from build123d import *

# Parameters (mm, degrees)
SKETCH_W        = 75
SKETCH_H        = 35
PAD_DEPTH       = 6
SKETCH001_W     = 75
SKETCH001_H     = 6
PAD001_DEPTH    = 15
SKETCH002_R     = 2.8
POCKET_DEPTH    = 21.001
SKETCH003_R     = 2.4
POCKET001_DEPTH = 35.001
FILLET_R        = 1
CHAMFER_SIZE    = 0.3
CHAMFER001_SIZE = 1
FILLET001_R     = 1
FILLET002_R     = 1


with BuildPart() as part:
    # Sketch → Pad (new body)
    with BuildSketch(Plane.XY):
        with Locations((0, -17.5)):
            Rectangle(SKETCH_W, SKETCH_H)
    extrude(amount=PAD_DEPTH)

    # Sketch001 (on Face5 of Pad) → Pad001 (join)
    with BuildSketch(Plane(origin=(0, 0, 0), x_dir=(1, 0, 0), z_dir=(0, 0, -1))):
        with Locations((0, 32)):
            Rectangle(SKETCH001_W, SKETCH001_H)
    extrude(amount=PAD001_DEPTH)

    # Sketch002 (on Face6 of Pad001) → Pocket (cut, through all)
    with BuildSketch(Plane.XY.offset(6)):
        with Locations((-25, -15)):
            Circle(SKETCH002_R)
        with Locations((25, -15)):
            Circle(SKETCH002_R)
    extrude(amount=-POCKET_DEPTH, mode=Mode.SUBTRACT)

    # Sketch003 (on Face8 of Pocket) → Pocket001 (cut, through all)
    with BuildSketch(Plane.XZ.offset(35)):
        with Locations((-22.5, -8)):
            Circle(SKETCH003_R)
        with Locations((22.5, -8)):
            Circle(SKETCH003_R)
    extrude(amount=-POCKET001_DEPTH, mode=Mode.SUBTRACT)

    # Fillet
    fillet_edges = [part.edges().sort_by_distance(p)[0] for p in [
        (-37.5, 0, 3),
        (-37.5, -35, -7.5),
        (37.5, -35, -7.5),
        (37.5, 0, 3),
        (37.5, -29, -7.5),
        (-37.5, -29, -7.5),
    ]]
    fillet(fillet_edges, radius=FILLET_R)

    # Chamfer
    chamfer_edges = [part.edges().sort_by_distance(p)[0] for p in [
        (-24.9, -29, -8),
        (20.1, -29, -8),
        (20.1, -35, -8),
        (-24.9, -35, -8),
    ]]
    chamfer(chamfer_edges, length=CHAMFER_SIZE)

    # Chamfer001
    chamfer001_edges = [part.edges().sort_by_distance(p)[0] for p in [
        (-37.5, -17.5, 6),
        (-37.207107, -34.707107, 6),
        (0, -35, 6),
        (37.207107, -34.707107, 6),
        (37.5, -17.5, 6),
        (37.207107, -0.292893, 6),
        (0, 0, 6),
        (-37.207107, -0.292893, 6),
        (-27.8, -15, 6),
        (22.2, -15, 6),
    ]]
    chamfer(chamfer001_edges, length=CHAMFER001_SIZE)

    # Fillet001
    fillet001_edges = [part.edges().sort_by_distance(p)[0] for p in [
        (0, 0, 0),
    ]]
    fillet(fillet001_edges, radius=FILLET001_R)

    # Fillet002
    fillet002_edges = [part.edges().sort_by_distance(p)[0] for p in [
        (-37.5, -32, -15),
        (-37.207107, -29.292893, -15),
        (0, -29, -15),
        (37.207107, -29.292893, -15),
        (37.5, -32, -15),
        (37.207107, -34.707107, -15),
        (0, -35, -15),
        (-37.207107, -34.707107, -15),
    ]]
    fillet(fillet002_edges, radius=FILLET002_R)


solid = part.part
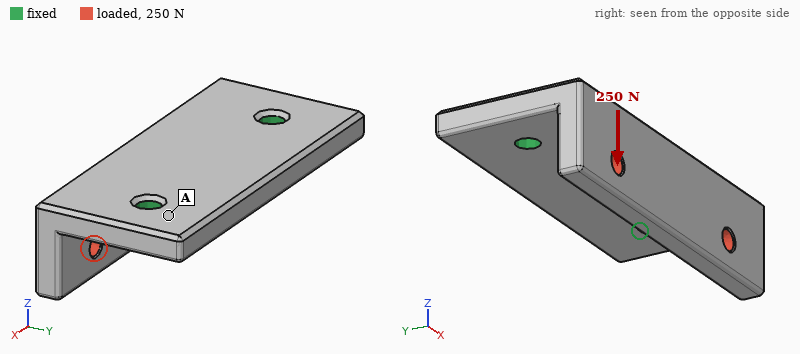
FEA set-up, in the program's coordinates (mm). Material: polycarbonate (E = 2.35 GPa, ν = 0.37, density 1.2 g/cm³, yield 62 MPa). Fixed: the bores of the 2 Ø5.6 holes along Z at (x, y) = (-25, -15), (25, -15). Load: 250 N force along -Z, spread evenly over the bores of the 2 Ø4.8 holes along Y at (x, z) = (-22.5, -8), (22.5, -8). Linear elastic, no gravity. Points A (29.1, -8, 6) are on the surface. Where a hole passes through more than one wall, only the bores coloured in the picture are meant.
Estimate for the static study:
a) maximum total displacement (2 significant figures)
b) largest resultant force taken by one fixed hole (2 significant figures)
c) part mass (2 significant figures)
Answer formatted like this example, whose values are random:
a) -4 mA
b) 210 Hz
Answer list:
a) 0.36 mm
b) 130 N
c) 26 g
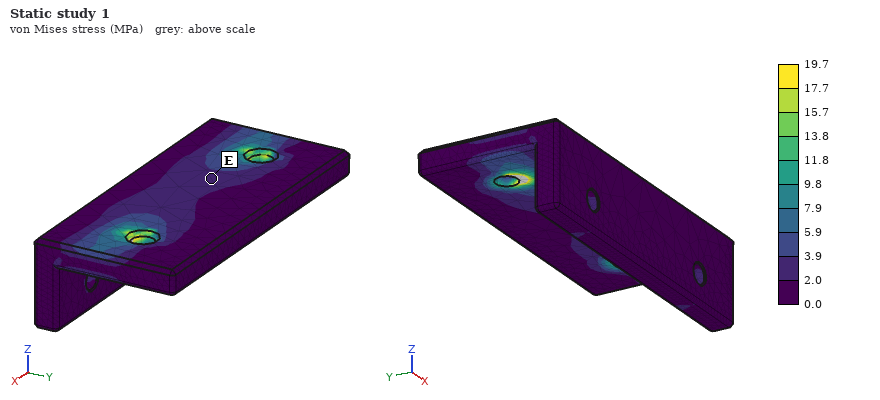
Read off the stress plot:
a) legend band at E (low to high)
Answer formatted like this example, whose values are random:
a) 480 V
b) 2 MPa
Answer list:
a) 2.0 to 3.9 MPa
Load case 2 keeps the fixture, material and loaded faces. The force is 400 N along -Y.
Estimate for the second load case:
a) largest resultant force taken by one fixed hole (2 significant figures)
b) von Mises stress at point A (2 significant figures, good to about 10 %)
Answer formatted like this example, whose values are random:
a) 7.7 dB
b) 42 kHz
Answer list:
a) 200 N
b) 2.3 MPa
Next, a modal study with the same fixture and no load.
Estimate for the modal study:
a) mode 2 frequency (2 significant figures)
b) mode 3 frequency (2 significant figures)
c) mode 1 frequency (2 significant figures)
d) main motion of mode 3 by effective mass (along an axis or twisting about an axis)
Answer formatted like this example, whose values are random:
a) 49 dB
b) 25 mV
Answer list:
a) 1900 Hz
b) 2900 Hz
c) 1300 Hz
d) along Z
